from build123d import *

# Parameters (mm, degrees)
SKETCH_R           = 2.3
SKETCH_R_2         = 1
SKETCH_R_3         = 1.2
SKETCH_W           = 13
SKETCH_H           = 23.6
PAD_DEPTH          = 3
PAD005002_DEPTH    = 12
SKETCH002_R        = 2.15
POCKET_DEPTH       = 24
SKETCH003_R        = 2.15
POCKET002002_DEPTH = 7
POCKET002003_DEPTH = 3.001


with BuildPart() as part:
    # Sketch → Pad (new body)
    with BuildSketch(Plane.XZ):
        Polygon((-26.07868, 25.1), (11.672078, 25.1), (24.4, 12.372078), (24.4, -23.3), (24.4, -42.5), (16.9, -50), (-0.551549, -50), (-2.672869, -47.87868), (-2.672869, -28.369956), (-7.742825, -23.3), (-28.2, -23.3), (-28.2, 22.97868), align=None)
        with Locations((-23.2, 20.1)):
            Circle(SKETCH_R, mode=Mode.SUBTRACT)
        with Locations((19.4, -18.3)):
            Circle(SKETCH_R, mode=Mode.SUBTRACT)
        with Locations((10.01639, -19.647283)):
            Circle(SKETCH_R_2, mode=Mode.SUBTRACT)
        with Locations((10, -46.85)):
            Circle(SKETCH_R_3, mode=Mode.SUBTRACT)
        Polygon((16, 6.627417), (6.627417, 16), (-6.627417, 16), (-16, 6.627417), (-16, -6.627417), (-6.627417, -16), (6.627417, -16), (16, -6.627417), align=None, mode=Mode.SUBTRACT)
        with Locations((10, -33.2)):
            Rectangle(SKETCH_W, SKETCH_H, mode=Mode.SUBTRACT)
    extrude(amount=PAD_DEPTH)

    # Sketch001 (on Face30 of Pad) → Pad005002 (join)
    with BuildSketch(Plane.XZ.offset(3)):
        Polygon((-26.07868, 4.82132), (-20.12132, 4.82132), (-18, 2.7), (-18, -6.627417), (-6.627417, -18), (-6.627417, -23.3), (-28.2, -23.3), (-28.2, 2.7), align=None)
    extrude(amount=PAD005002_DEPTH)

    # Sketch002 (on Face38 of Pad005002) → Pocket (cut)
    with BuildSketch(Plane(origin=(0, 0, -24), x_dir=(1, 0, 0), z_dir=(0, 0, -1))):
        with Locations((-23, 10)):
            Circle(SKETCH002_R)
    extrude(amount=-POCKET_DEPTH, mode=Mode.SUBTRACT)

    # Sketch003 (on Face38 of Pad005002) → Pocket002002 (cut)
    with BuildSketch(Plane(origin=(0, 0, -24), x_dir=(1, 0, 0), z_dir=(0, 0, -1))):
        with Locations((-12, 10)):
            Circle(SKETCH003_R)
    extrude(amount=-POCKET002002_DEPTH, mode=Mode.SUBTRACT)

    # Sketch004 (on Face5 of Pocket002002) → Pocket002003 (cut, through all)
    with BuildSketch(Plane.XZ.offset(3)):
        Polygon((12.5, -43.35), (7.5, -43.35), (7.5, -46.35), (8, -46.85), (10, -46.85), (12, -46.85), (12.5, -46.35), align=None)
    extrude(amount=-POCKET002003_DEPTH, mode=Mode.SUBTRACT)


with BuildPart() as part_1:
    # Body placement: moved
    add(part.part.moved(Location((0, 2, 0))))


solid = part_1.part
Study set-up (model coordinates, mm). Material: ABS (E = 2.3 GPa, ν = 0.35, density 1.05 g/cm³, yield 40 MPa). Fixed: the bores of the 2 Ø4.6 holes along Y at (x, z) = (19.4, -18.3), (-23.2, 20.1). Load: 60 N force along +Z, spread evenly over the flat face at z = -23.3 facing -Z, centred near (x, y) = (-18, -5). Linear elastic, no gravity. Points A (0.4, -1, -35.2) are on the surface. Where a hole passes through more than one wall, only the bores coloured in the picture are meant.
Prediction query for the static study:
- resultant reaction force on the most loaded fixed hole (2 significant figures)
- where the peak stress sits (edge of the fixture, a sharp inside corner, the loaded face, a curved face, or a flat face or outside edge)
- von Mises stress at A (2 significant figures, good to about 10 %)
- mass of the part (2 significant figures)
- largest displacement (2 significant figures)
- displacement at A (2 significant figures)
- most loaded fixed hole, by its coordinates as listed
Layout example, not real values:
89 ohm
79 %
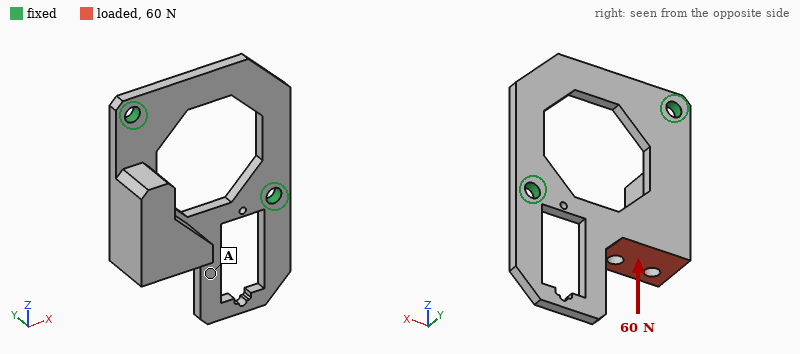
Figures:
54 N
a curved face
1.4 MPa
11 g
0.98 mm
0.47 mm
(-23.2, 20.1)
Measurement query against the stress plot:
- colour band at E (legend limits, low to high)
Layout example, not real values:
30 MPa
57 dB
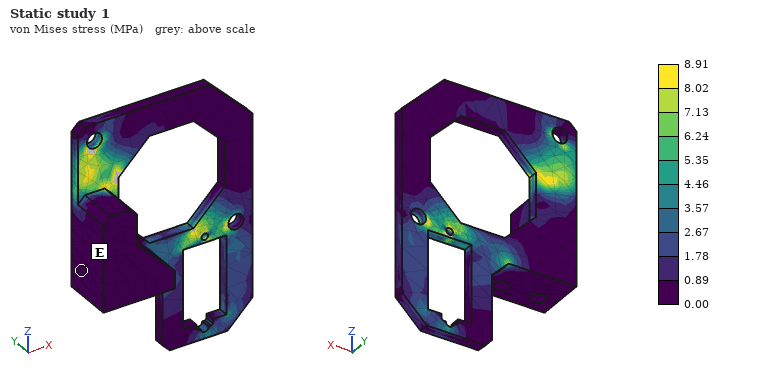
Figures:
0.00 to 0.89 MPa
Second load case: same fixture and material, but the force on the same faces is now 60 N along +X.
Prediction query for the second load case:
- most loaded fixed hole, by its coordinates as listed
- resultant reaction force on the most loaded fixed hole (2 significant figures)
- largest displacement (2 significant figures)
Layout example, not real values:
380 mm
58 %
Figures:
(19.4, -18.3)
56 N
0.94 mm
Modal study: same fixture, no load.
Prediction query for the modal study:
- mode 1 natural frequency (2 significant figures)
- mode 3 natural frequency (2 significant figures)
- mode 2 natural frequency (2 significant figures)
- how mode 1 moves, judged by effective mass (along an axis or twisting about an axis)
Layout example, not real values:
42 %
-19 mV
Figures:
310 Hz
760 Hz
710 Hz
along Y
